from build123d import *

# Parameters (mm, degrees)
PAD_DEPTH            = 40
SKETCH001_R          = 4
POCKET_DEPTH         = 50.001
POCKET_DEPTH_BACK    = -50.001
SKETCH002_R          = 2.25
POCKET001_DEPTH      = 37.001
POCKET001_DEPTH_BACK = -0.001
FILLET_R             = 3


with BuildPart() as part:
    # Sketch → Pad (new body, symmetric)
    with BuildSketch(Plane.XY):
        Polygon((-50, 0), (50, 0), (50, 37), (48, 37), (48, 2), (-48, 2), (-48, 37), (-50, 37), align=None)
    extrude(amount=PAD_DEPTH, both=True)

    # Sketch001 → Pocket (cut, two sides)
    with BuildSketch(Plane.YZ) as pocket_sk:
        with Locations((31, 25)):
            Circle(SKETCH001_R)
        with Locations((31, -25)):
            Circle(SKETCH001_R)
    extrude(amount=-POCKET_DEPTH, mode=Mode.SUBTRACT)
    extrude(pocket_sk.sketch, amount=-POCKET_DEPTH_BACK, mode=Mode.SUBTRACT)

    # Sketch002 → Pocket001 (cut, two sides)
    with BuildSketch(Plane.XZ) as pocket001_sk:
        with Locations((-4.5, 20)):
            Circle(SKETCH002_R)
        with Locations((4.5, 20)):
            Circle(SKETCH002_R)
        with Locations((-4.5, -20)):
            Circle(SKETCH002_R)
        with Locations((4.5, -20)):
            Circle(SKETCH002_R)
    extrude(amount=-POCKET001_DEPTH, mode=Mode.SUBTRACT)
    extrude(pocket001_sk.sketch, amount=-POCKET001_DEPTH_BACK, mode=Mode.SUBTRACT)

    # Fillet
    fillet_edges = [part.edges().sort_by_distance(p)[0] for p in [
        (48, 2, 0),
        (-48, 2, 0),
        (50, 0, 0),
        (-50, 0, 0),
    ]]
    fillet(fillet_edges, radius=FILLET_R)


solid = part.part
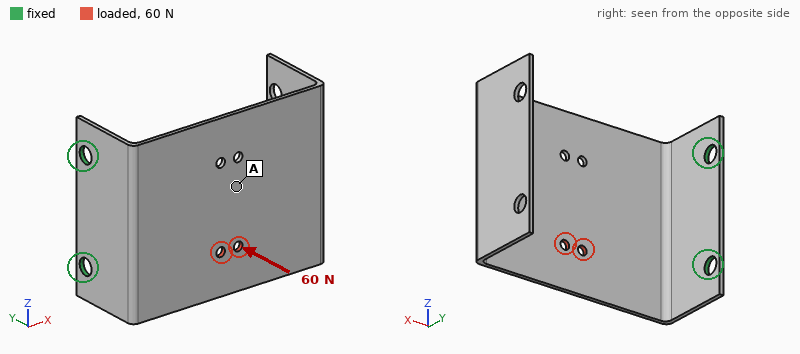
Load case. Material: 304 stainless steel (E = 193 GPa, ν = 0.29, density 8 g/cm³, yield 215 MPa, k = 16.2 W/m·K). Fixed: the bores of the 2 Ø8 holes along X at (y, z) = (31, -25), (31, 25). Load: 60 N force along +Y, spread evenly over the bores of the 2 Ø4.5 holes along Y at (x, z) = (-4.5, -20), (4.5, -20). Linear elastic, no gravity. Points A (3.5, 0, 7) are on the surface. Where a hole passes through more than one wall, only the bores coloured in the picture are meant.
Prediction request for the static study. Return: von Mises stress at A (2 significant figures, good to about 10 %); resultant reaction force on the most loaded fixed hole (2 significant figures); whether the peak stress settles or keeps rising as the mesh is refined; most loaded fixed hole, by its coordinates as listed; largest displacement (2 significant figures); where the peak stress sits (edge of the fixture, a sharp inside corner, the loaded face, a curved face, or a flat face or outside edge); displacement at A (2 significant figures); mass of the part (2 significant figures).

8.4 MPa
54 N
keeps rising
(31, -25)
1.4 mm
edge of the fixture
0.60 mm
210 g
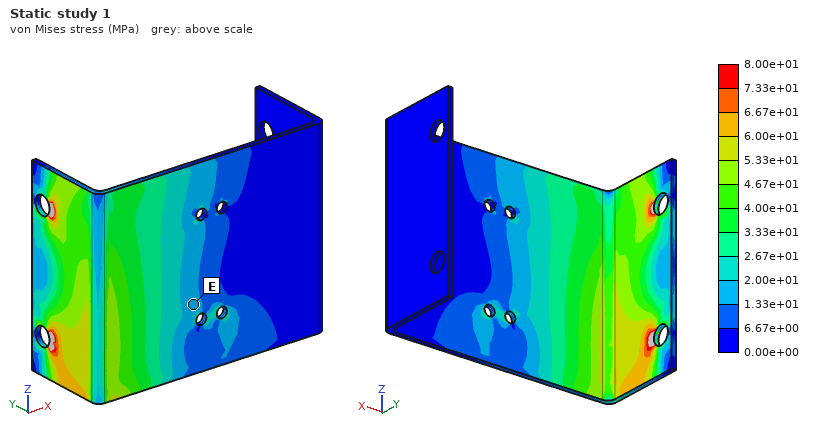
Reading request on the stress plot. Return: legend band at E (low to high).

1.33e+01 to 2.00e+01 MPa
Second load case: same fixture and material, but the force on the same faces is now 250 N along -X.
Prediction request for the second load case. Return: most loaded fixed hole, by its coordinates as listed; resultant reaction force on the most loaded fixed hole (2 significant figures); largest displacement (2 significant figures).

(31, -25)
210 N
1.1 mm
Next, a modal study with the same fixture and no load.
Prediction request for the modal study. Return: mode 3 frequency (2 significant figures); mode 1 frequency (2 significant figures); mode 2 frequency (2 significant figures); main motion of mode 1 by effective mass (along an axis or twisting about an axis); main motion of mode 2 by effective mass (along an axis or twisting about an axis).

370 Hz
77 Hz
200 Hz
along Y
along Z
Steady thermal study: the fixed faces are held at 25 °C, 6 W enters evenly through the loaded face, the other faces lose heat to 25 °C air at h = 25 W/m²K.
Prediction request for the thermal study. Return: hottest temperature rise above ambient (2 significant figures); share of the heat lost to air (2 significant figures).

72 K
96 %
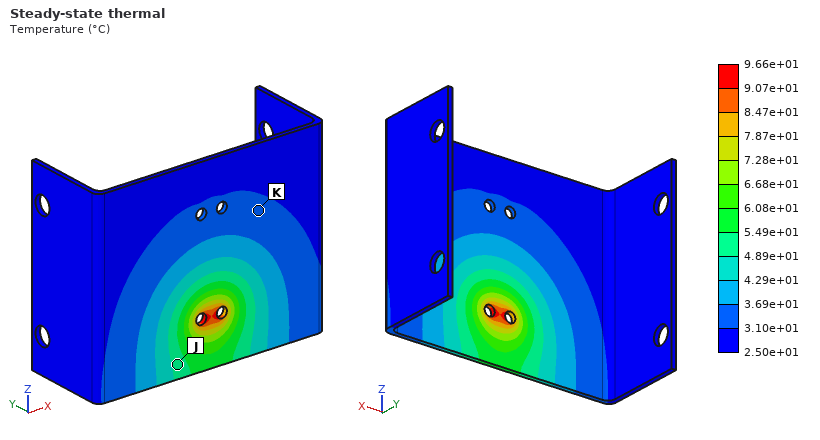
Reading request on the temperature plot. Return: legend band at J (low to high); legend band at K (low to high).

4.89e+01 to 5.49e+01 °C
3.10e+01 to 3.69e+01 °C
